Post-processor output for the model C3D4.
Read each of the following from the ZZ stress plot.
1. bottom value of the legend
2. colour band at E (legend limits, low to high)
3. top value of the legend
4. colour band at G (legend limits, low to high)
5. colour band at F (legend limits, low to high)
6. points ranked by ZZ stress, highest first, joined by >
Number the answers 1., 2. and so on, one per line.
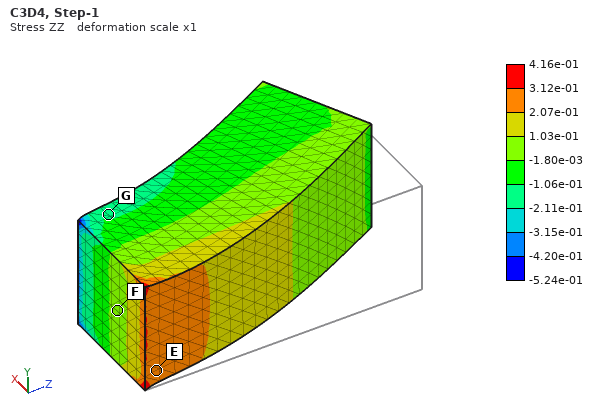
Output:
1. -5.24e-01
2. 2.07e-01 to 3.12e-01
3. 4.16e-01
4. -2.11e-01 to -1.06e-01
5. -1.80e-03 to 1.03e-01
6. E > F > G
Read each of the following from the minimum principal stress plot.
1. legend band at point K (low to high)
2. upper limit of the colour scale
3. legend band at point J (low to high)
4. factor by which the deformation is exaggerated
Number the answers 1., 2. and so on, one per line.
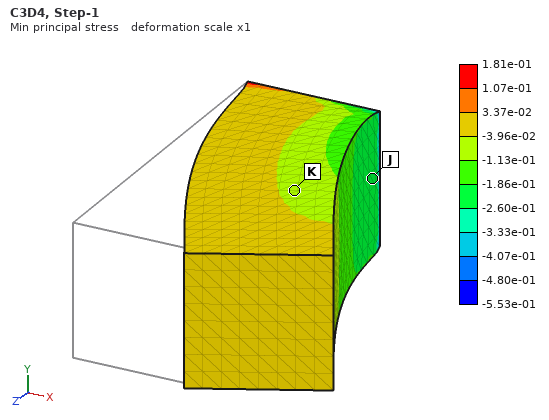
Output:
1. -1.13e-01 to -3.96e-02
2. 1.81e-01
3. -2.60e-01 to -1.86e-01
4. 1
